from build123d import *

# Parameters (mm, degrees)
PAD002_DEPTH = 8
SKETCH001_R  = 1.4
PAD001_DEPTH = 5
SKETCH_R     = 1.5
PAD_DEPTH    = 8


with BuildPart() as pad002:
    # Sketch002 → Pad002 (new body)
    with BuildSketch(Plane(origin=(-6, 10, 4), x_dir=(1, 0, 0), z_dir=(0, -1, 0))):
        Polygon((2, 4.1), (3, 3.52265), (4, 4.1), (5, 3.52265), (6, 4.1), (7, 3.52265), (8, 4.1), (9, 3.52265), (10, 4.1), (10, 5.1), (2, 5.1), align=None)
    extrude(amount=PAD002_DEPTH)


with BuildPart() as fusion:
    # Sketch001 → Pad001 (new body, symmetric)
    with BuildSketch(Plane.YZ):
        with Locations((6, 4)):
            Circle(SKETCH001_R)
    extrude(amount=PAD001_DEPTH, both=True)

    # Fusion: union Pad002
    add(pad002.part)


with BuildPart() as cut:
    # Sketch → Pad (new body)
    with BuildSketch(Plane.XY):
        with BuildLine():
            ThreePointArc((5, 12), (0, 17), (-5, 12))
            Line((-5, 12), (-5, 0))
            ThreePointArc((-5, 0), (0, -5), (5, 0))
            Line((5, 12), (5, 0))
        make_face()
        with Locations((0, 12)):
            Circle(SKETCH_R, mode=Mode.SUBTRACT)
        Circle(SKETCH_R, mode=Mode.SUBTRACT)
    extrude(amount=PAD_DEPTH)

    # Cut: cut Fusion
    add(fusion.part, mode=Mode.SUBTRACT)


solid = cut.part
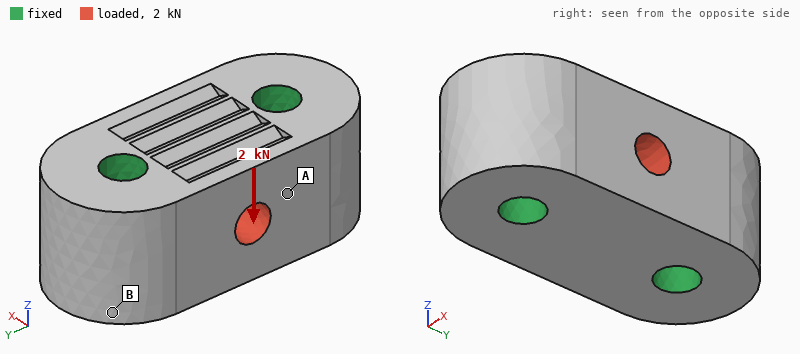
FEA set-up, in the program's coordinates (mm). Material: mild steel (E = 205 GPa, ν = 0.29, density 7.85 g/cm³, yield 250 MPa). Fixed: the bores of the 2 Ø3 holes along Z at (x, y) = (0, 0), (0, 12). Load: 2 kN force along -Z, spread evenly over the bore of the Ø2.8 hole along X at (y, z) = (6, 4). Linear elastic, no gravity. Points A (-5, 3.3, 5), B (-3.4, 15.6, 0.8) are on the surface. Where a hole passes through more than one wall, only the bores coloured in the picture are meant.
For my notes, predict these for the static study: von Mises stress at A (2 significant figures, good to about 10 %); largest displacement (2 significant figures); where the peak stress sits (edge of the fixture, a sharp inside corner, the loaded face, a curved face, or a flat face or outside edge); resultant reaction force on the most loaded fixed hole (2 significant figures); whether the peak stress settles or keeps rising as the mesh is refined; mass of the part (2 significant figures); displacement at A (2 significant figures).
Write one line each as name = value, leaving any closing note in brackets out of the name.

von Mises stress at A = 23 MPa
largest displacement = 1.3 µm
where the peak stress sits = edge of the fixture
resultant reaction force on the most loaded fixed hole = 1.0 kN
whether the peak stress settles or keeps rising as the mesh is refined = keeps rising
mass of the part = 11 g
displacement at A = 0.78 µm
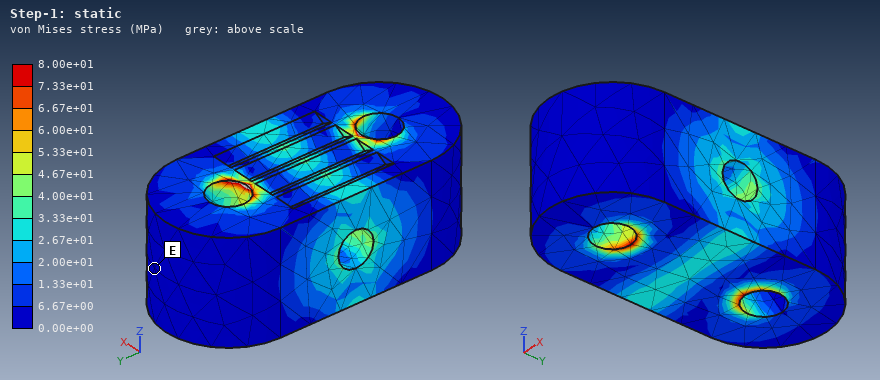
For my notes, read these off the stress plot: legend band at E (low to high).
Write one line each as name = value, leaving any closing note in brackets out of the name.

legend band at E = 0.00e+00 to 6.67e+00 MPa
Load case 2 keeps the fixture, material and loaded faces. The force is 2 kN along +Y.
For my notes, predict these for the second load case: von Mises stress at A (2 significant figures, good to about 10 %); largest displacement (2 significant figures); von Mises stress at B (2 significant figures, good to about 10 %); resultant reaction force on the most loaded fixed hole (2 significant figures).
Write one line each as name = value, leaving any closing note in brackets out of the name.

von Mises stress at A = 17 MPa
largest displacement = 0.54 µm
von Mises stress at B = 4.0 MPa
resultant reaction force on the most loaded fixed hole = 1.0 kN
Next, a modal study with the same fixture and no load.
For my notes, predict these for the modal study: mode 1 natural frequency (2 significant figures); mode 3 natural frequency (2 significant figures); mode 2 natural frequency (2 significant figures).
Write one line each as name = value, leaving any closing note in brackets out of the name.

mode 1 natural frequency = 110 kHz
mode 3 natural frequency = 120 kHz
mode 2 natural frequency = 120 kHz
